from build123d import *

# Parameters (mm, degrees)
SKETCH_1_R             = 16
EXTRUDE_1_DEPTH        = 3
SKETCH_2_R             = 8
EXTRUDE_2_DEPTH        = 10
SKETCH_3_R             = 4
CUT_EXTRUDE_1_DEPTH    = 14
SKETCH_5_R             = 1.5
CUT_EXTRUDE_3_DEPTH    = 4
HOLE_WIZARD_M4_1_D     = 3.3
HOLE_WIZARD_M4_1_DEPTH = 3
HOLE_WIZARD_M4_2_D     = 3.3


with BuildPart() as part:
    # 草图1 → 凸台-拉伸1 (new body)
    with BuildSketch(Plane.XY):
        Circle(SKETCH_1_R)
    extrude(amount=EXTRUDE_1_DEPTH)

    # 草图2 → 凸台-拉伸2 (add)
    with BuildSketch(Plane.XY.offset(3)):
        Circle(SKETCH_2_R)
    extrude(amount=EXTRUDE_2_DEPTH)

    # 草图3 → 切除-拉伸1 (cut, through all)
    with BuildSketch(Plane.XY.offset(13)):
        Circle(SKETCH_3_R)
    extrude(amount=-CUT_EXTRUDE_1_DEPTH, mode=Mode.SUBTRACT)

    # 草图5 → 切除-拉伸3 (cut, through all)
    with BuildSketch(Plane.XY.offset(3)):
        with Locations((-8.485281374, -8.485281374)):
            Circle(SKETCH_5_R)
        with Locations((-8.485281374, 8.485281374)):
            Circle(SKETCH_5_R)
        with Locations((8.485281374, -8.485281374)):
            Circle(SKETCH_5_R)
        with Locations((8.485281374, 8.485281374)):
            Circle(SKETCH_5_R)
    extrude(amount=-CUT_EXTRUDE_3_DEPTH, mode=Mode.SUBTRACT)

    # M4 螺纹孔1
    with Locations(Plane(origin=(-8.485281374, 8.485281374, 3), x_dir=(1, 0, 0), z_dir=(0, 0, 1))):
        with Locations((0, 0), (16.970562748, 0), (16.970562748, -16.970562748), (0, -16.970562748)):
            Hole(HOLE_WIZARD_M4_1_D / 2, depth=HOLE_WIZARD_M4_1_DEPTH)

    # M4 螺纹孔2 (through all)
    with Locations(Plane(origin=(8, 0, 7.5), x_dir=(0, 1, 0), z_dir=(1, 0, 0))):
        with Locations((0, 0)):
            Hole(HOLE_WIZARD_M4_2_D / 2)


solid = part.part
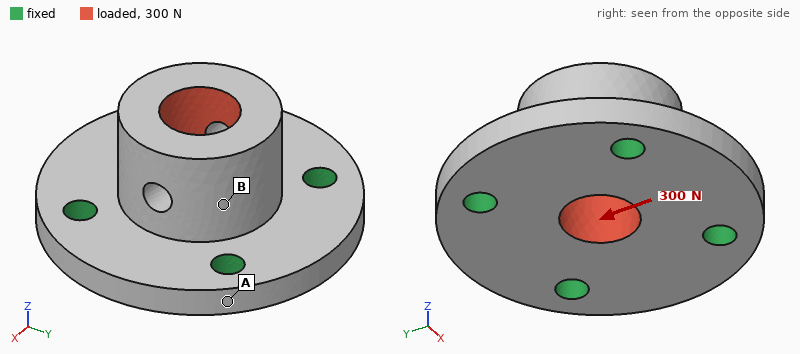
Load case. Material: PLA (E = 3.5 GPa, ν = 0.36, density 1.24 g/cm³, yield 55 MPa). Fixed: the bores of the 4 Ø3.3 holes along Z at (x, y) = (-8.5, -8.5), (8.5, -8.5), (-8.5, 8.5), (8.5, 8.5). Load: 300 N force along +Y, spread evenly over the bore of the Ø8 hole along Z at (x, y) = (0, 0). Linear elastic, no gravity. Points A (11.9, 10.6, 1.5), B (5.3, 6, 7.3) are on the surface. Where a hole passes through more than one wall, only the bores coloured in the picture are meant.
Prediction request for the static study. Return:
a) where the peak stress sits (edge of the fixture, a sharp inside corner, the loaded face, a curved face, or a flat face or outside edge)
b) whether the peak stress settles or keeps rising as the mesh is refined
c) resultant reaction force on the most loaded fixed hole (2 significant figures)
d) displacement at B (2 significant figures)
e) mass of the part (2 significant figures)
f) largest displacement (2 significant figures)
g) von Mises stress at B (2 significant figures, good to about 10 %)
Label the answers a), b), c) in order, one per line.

a) edge of the fixture
b) keeps rising
c) 92 N
d) 25 µm
e) 4.5 g
f) 44 µm
g) 2.0 MPa
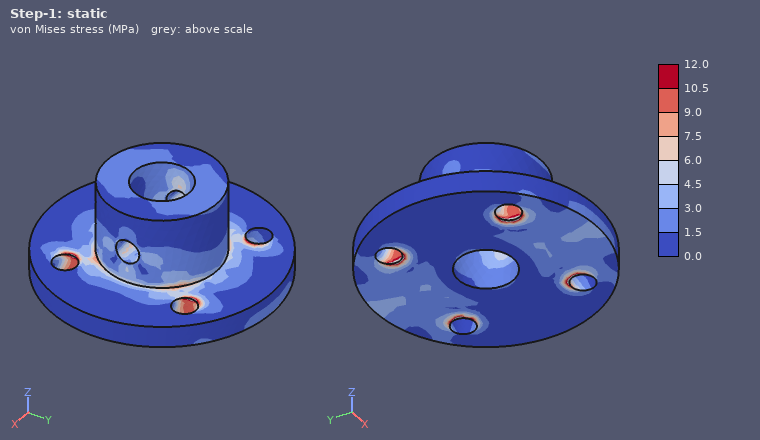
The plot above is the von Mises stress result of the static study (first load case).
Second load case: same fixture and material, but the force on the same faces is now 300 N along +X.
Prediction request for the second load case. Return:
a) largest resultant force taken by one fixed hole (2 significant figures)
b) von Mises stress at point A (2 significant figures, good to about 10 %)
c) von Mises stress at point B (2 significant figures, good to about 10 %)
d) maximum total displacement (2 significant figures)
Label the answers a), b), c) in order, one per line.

a) 92 N
b) 1.1 MPa
c) 1.4 MPa
d) 41 µm
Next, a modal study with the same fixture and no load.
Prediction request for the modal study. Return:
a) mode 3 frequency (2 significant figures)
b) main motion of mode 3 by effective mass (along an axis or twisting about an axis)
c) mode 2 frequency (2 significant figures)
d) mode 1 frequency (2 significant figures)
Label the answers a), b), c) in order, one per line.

a) 12 kHz
b) along Z
c) 9900 Hz
d) 9600 Hz
